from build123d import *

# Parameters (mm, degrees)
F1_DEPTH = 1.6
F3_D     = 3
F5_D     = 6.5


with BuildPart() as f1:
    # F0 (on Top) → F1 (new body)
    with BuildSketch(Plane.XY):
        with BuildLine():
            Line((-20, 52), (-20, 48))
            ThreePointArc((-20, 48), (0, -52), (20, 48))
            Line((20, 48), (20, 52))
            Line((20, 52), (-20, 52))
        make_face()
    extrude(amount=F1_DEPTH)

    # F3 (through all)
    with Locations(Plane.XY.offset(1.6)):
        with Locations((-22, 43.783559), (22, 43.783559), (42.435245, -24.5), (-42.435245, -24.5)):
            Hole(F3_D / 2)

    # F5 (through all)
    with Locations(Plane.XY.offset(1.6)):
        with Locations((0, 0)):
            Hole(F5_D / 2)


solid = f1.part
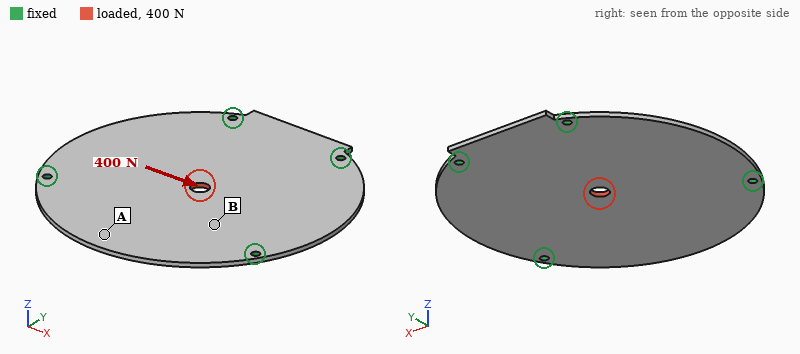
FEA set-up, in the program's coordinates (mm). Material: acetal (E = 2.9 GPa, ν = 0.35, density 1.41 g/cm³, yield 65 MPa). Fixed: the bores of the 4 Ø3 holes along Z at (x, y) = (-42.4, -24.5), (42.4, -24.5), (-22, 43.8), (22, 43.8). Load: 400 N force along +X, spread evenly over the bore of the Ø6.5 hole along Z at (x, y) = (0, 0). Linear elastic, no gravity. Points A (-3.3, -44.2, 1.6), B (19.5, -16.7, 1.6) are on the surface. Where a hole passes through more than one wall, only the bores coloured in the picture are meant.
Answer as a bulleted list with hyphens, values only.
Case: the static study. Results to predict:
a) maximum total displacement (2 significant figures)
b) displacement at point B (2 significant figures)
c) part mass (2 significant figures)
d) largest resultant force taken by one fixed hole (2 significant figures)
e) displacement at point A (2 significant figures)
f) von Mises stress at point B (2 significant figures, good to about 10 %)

- 97 µm
- 42 µm
- 19 g
- 130 N
- 26 µm
- 3.5 MPa
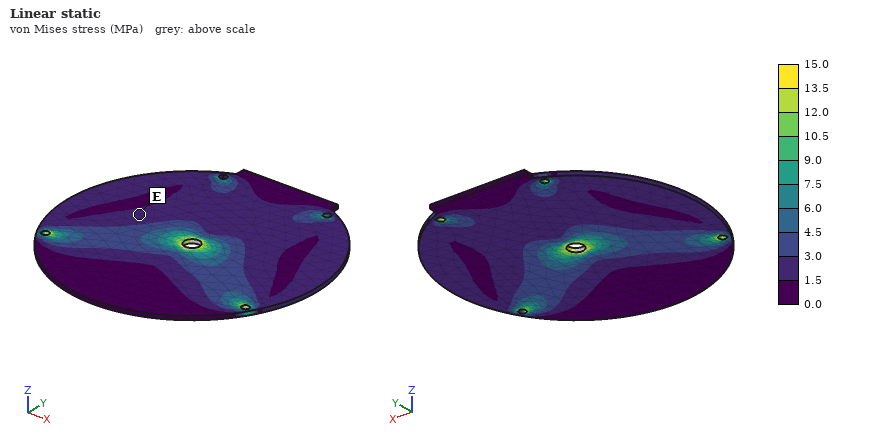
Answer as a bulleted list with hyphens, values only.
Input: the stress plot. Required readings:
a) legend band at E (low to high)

- 1.5 to 3.0 MPa
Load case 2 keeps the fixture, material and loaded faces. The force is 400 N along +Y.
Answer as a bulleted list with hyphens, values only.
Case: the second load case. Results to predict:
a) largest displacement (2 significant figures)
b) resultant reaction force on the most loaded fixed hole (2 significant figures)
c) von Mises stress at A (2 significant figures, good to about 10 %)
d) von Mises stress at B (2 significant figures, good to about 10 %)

- 98 µm
- 110 N
- 1.8 MPa
- 2.3 MPa
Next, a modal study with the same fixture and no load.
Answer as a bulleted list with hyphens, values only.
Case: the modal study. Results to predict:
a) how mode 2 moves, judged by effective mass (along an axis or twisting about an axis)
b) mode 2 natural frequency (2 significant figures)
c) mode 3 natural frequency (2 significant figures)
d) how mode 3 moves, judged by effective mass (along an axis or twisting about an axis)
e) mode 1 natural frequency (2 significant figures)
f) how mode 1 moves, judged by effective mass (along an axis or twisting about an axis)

- along Z
- 340 Hz
- 410 Hz
- twisting about Y
- 250 Hz
- along Z
